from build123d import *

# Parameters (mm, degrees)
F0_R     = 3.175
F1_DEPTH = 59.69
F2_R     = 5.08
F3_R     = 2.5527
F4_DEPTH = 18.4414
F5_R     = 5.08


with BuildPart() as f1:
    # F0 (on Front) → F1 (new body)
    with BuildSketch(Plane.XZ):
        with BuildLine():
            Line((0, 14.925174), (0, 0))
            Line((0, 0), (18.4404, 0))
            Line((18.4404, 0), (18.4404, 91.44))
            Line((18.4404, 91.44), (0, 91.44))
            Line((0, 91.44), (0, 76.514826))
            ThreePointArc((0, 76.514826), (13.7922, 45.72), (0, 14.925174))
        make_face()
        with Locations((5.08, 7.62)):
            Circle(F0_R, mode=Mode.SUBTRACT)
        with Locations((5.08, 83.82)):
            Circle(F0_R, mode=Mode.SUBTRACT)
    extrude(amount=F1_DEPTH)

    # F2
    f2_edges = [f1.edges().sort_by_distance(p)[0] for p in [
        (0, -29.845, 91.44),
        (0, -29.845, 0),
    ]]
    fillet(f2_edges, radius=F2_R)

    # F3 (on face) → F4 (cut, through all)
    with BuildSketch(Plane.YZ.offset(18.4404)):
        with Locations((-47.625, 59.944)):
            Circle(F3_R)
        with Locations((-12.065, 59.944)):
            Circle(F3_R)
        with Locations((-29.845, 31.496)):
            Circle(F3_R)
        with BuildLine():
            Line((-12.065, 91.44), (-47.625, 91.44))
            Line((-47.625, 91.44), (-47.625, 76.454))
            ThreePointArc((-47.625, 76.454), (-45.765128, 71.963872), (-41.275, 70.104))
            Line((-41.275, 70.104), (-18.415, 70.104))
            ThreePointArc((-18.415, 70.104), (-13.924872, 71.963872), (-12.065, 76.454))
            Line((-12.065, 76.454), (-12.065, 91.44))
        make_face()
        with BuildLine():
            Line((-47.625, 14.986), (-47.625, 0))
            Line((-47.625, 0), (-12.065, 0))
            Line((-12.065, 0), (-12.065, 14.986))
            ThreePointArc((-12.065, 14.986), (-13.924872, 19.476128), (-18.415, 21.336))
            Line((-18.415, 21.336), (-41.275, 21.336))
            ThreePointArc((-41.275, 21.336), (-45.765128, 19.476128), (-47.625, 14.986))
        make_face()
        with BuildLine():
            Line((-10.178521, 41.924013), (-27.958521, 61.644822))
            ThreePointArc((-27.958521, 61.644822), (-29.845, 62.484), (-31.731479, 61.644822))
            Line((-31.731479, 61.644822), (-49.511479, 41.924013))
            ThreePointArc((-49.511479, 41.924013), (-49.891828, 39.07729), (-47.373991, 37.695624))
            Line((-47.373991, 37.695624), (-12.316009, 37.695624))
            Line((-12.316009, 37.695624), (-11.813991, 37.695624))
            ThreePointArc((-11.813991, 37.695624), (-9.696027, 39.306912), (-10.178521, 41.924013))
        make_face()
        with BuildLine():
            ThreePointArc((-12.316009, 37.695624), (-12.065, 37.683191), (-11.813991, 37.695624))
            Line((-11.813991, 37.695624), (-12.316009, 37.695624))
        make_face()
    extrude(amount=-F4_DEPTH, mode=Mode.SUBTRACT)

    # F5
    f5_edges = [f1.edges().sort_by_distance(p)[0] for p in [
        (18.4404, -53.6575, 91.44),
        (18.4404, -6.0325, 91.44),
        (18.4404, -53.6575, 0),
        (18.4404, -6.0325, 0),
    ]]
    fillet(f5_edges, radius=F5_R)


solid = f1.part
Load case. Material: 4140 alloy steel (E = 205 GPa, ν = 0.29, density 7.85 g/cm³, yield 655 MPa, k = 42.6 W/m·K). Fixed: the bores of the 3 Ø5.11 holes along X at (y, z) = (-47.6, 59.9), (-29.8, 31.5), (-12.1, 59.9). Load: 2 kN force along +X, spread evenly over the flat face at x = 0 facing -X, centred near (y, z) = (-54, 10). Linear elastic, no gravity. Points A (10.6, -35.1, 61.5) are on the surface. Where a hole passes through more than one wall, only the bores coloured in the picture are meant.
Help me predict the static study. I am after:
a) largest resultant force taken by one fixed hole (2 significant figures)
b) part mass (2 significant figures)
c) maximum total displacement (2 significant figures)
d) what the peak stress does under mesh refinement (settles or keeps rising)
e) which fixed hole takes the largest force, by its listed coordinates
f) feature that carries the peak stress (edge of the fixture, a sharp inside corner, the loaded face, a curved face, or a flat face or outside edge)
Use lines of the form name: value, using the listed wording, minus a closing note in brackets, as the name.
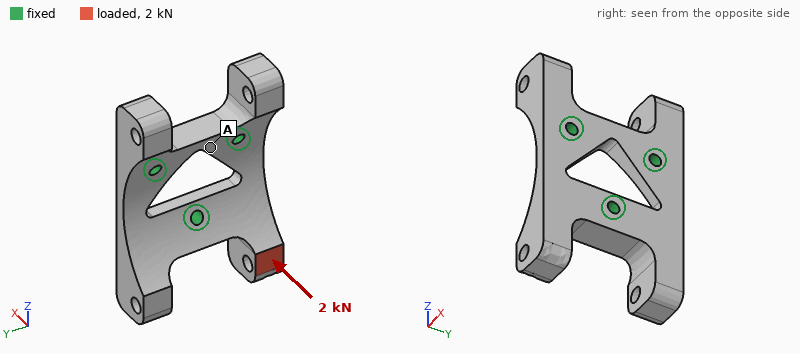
largest resultant force taken by one fixed hole: 2.3 kN
part mass: 270 g
maximum total displacement: 0.21 mm
what the peak stress does under mesh refinement: keeps rising
which fixed hole takes the largest force, by its listed coordinates: (-29.8, 31.5)
feature that carries the peak stress: edge of the fixture
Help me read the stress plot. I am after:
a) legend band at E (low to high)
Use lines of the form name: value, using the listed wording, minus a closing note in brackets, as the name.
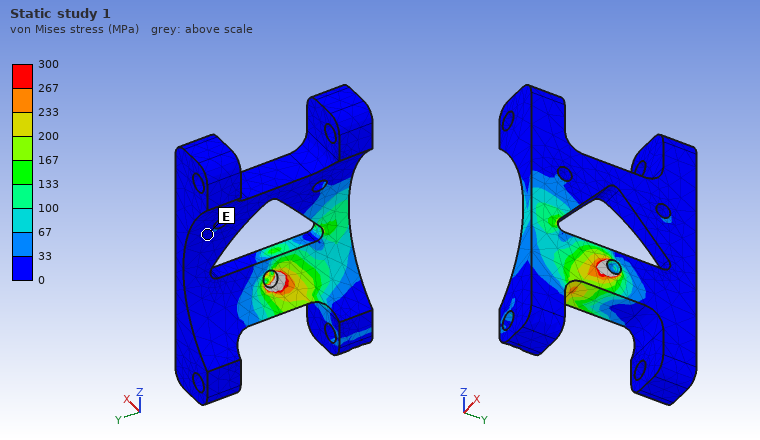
legend band at E: 0 to 33 MPa
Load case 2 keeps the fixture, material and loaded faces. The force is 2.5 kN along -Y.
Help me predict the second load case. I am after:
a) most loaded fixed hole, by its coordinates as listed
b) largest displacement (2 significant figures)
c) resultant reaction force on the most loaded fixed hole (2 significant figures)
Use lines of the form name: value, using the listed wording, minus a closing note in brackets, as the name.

most loaded fixed hole, by its coordinates as listed: (-29.8, 31.5)
largest displacement: 90 µm
resultant reaction force on the most loaded fixed hole: 3.4 kN
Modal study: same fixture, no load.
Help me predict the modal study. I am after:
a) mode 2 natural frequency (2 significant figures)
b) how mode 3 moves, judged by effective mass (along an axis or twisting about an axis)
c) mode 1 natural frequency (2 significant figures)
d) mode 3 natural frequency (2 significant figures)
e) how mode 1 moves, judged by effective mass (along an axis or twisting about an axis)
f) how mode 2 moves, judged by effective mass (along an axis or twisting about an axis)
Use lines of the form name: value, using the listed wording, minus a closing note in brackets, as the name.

mode 2 natural frequency: 3400 Hz
how mode 3 moves, judged by effective mass: along X
mode 1 natural frequency: 3000 Hz
mode 3 natural frequency: 6000 Hz
how mode 1 moves, judged by effective mass: twisting about Z
how mode 2 moves, judged by effective mass: along X
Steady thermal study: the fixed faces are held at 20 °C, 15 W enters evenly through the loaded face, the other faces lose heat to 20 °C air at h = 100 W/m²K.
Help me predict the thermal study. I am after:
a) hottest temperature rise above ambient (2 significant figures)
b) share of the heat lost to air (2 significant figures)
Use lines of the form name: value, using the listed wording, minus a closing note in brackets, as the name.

hottest temperature rise above ambient: 62 K
share of the heat lost to air: 55 %
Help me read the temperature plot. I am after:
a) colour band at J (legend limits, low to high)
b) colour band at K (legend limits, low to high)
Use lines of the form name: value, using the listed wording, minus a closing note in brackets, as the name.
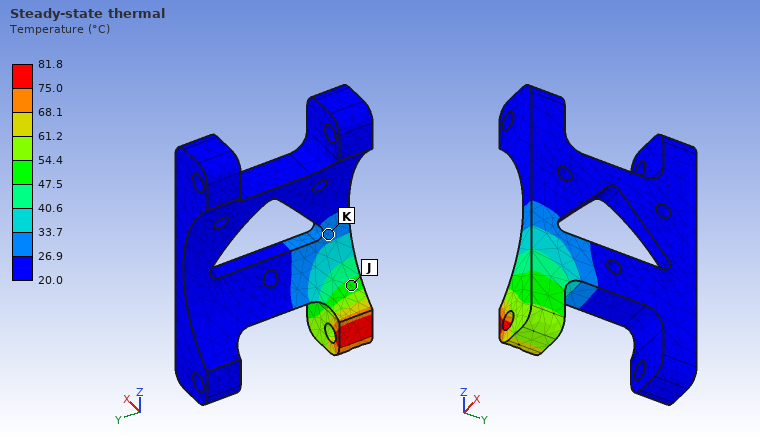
colour band at J: 47.5 to 54.4 °C
colour band at K: 26.9 to 33.7 °C
